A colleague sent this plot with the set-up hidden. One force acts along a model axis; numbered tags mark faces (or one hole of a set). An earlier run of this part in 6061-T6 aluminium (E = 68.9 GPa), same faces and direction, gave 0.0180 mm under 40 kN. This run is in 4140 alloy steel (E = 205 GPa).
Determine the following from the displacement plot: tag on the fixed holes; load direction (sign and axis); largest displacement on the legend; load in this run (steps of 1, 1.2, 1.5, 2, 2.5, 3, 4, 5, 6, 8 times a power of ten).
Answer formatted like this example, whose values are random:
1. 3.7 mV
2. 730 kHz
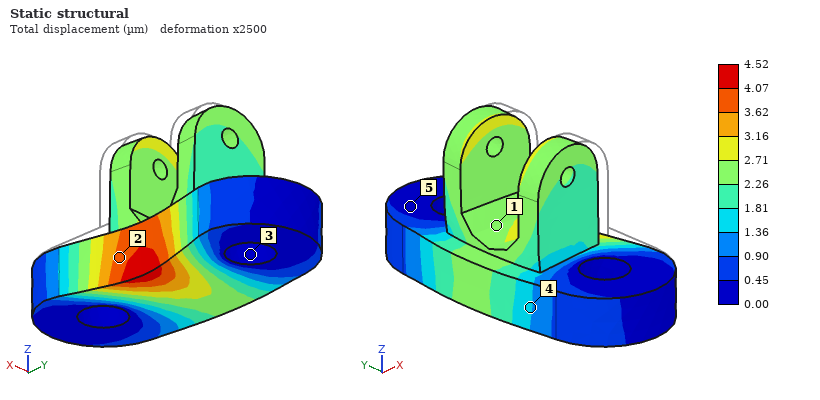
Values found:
1. 3
2. -X
3. 4.52 µm
4. 30 kN
